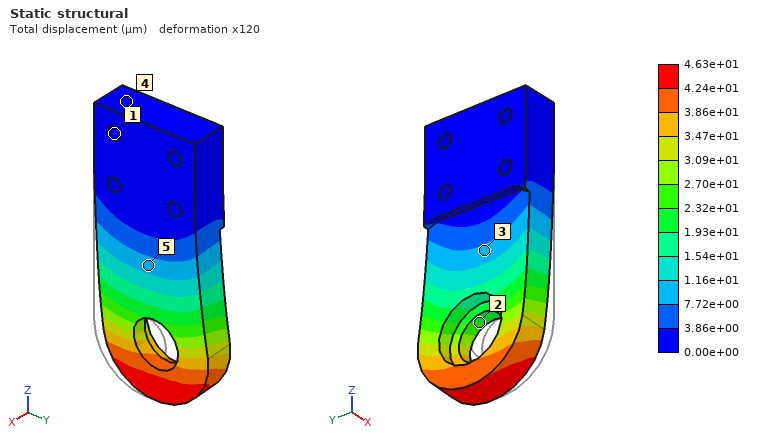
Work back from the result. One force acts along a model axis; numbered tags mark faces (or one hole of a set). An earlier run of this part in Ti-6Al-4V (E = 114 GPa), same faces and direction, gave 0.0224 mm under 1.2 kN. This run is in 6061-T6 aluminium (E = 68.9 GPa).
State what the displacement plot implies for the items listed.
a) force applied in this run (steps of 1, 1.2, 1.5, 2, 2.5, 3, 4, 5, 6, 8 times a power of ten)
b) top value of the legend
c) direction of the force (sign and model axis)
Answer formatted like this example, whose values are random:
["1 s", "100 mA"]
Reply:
["1.5 kN", "4.63e+01 µm", "+Y"]
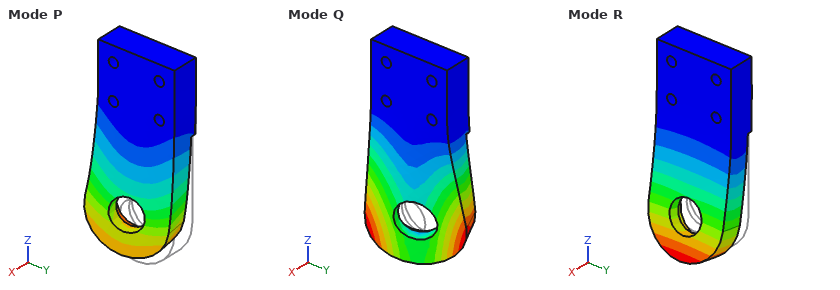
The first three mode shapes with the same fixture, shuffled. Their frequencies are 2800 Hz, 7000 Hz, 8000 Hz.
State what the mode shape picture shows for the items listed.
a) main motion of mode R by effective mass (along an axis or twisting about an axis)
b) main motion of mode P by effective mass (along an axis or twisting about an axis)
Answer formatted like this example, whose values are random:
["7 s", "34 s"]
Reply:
["along X", "along Y"]
